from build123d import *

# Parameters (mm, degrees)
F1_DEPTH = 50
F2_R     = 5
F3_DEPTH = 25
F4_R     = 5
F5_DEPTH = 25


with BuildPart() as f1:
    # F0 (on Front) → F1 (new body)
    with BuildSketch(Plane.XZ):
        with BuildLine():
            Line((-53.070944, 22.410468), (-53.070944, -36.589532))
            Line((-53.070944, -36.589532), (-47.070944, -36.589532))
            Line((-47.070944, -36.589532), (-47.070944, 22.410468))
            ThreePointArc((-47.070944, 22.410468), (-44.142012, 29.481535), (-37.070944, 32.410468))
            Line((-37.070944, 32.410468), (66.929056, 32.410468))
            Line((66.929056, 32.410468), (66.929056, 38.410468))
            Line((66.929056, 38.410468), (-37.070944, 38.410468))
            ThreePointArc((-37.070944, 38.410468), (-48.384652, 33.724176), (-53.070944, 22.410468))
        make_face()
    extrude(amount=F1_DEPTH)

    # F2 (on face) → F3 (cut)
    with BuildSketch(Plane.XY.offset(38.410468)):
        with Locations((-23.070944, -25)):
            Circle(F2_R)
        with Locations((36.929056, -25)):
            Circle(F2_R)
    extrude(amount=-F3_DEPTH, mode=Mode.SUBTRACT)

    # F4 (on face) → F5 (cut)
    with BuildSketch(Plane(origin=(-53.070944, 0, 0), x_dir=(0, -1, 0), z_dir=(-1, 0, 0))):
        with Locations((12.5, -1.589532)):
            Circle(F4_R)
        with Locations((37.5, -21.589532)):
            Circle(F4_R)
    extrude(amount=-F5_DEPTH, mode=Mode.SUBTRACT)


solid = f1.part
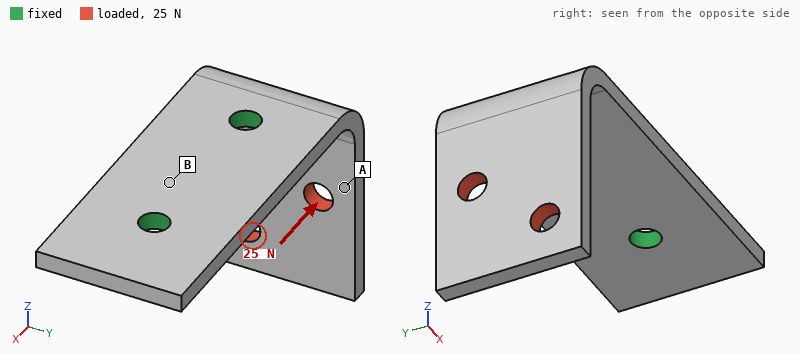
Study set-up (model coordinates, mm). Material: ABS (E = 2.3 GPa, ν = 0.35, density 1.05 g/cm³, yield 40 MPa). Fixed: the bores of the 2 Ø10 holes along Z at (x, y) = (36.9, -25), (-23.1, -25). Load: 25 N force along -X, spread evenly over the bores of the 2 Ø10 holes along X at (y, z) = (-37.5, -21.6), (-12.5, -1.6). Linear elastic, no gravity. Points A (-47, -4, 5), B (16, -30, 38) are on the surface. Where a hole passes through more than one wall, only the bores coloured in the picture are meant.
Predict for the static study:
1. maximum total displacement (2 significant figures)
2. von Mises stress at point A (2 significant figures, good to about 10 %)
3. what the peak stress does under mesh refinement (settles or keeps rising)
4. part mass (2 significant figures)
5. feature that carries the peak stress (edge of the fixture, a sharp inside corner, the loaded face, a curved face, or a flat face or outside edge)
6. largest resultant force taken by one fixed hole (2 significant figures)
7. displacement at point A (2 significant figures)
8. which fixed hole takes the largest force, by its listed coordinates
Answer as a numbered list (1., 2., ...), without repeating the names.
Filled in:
1. 1.6 mm
2. 1.4 MPa
3. keeps rising
4. 56 g
5. edge of the fixture
6. 23 N
7. 0.52 mm
8. (-23.1, -25)
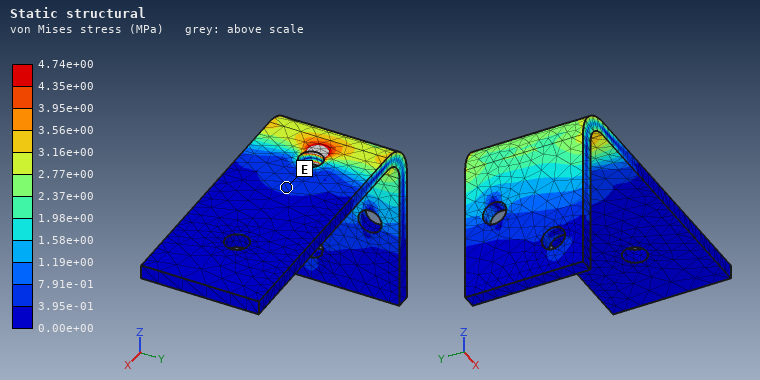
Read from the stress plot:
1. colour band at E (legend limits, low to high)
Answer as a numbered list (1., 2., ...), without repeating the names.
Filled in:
1. 3.95e-01 to 7.91e-01 MPa
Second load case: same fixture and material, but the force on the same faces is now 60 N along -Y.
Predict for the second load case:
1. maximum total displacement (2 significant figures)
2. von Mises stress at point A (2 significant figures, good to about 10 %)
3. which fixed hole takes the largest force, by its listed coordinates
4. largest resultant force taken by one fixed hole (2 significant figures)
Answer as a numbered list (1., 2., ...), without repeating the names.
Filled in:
1. 1.4 mm
2. 1.2 MPa
3. (-23.1, -25)
4. 78 N
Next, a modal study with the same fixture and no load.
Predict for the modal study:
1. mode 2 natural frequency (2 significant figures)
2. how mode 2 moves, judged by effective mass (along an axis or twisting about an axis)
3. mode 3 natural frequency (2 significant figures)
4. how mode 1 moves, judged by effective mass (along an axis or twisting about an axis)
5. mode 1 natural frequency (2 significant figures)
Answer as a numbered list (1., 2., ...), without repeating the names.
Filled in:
1. 310 Hz
2. along Y
3. 820 Hz
4. along X
5. 190 Hz
